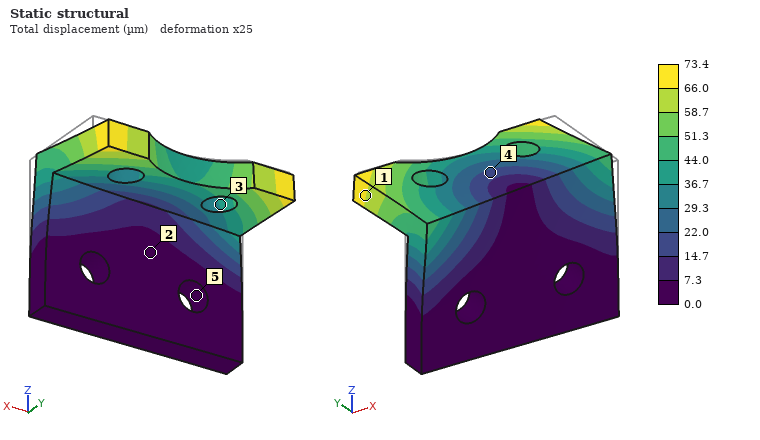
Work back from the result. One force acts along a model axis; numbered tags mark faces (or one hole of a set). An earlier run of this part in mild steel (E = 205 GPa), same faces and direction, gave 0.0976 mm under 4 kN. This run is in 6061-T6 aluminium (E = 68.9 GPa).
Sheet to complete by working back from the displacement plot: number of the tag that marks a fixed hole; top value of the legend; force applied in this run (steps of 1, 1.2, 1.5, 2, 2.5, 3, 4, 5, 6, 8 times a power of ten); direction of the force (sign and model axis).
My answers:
5
73.4 µm
1 kN
-X
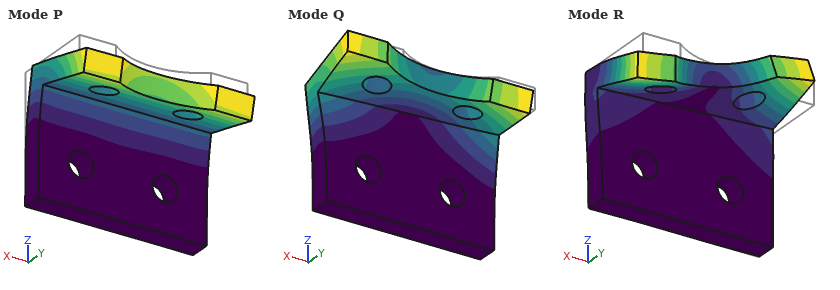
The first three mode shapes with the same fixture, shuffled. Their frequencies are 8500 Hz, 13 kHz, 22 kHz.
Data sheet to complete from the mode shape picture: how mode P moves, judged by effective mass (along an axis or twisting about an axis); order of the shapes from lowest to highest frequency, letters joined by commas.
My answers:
along Y
P, Q, R
